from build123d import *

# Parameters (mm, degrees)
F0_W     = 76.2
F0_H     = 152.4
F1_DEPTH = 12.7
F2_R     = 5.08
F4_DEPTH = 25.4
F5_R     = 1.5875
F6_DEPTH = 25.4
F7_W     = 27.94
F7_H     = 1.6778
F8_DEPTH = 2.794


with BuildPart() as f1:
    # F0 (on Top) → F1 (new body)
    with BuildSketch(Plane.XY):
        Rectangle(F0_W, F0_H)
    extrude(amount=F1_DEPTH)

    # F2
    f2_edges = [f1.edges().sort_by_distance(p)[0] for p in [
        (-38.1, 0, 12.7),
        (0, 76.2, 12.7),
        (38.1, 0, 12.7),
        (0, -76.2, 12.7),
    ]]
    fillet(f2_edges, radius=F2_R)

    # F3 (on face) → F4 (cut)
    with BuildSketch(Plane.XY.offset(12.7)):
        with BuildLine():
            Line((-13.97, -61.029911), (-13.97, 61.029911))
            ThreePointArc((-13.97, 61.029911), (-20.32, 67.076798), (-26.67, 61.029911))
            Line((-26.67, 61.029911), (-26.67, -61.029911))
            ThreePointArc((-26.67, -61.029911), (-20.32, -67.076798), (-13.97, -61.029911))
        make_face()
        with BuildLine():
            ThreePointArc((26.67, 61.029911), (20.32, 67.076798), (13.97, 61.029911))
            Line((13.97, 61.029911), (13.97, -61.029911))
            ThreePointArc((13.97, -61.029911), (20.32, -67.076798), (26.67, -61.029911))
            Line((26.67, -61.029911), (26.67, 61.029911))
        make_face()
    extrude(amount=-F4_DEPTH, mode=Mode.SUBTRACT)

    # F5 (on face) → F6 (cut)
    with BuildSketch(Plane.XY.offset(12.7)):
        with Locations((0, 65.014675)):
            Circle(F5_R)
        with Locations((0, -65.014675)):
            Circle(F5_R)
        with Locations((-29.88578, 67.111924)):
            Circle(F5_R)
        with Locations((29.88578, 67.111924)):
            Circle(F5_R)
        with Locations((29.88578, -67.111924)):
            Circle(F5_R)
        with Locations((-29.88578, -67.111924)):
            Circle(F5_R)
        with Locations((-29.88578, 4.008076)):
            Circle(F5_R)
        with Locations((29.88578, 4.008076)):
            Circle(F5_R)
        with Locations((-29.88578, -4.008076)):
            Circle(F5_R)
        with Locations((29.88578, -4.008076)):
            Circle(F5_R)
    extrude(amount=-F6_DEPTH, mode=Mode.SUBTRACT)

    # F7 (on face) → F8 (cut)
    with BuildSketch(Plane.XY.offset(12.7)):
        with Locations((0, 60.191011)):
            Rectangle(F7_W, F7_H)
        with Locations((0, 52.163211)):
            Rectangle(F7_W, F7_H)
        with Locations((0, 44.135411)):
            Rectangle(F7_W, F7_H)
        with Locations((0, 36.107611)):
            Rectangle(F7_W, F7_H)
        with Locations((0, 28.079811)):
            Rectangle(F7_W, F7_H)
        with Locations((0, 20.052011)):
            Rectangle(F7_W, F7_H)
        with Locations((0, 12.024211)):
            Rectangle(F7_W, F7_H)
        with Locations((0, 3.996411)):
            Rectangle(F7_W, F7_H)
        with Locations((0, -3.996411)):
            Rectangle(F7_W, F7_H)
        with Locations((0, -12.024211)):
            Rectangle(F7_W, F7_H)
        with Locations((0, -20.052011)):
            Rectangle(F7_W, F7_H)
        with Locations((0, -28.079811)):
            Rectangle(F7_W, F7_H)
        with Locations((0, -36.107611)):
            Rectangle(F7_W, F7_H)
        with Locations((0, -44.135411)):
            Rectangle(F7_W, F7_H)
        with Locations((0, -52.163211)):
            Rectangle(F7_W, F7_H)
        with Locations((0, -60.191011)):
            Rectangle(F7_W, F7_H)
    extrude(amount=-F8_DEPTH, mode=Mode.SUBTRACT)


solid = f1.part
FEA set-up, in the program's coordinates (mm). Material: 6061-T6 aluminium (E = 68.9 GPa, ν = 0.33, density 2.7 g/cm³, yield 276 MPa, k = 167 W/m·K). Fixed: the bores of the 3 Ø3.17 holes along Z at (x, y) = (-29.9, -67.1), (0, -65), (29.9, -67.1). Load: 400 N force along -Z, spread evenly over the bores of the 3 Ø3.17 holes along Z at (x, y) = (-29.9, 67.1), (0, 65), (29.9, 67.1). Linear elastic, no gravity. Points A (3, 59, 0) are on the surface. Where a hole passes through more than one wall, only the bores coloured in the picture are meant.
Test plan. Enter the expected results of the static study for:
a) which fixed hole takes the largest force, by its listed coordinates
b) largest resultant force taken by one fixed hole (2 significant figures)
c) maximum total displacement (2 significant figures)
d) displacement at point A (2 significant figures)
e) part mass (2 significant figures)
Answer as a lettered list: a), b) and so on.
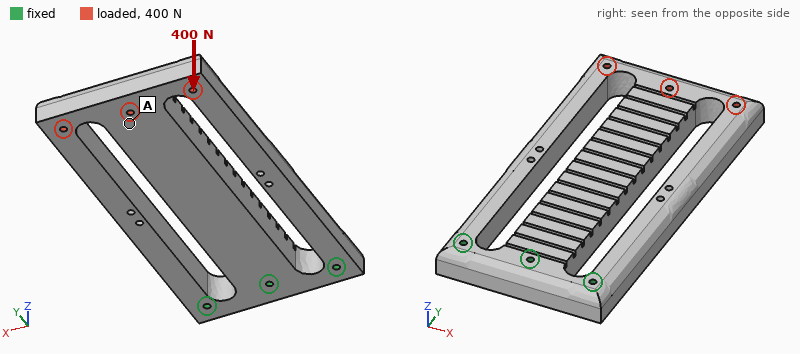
a) (0, -65)
b) 490 N
c) 0.83 mm
d) 0.68 mm
e) 270 g
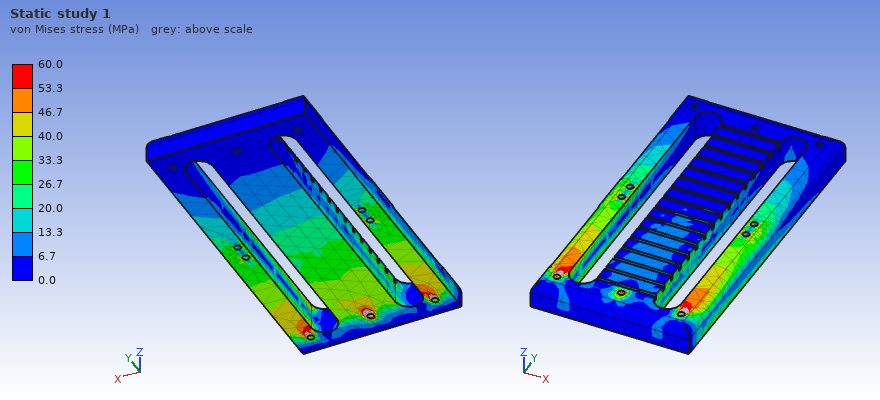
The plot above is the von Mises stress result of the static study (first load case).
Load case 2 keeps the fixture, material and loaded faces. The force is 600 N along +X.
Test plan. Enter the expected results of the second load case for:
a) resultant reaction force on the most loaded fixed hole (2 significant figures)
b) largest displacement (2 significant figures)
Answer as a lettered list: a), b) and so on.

a) 1.2 kN
b) 0.15 mm
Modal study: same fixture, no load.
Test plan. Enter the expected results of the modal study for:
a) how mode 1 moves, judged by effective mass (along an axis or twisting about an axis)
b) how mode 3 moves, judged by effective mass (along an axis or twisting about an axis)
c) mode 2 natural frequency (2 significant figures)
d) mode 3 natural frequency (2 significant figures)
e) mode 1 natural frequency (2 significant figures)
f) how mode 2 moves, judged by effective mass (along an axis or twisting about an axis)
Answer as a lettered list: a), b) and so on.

a) along Z
b) twisting about Y
c) 980 Hz
d) 1300 Hz
e) 410 Hz
f) along X
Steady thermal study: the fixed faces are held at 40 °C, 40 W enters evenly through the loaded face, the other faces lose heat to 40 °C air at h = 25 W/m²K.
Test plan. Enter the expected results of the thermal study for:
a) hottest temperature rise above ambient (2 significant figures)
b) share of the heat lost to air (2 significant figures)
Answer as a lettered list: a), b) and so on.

a) 43 K
b) 38 %
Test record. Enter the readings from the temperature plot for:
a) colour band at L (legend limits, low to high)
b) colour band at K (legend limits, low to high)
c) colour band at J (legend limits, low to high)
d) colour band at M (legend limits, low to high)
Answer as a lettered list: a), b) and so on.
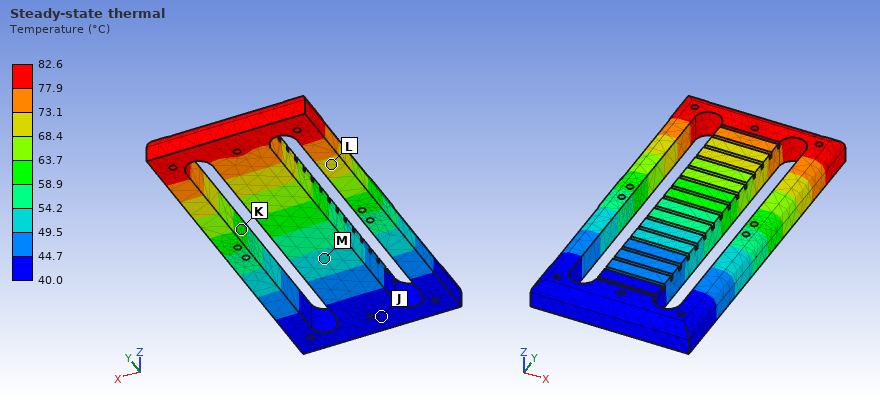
a) 68.4 to 73.1 °C
b) 58.9 to 63.7 °C
c) 40.0 to 44.7 °C
d) 49.5 to 54.2 °C
